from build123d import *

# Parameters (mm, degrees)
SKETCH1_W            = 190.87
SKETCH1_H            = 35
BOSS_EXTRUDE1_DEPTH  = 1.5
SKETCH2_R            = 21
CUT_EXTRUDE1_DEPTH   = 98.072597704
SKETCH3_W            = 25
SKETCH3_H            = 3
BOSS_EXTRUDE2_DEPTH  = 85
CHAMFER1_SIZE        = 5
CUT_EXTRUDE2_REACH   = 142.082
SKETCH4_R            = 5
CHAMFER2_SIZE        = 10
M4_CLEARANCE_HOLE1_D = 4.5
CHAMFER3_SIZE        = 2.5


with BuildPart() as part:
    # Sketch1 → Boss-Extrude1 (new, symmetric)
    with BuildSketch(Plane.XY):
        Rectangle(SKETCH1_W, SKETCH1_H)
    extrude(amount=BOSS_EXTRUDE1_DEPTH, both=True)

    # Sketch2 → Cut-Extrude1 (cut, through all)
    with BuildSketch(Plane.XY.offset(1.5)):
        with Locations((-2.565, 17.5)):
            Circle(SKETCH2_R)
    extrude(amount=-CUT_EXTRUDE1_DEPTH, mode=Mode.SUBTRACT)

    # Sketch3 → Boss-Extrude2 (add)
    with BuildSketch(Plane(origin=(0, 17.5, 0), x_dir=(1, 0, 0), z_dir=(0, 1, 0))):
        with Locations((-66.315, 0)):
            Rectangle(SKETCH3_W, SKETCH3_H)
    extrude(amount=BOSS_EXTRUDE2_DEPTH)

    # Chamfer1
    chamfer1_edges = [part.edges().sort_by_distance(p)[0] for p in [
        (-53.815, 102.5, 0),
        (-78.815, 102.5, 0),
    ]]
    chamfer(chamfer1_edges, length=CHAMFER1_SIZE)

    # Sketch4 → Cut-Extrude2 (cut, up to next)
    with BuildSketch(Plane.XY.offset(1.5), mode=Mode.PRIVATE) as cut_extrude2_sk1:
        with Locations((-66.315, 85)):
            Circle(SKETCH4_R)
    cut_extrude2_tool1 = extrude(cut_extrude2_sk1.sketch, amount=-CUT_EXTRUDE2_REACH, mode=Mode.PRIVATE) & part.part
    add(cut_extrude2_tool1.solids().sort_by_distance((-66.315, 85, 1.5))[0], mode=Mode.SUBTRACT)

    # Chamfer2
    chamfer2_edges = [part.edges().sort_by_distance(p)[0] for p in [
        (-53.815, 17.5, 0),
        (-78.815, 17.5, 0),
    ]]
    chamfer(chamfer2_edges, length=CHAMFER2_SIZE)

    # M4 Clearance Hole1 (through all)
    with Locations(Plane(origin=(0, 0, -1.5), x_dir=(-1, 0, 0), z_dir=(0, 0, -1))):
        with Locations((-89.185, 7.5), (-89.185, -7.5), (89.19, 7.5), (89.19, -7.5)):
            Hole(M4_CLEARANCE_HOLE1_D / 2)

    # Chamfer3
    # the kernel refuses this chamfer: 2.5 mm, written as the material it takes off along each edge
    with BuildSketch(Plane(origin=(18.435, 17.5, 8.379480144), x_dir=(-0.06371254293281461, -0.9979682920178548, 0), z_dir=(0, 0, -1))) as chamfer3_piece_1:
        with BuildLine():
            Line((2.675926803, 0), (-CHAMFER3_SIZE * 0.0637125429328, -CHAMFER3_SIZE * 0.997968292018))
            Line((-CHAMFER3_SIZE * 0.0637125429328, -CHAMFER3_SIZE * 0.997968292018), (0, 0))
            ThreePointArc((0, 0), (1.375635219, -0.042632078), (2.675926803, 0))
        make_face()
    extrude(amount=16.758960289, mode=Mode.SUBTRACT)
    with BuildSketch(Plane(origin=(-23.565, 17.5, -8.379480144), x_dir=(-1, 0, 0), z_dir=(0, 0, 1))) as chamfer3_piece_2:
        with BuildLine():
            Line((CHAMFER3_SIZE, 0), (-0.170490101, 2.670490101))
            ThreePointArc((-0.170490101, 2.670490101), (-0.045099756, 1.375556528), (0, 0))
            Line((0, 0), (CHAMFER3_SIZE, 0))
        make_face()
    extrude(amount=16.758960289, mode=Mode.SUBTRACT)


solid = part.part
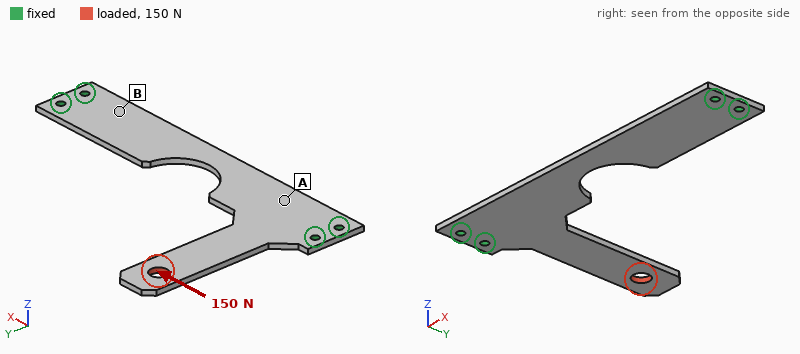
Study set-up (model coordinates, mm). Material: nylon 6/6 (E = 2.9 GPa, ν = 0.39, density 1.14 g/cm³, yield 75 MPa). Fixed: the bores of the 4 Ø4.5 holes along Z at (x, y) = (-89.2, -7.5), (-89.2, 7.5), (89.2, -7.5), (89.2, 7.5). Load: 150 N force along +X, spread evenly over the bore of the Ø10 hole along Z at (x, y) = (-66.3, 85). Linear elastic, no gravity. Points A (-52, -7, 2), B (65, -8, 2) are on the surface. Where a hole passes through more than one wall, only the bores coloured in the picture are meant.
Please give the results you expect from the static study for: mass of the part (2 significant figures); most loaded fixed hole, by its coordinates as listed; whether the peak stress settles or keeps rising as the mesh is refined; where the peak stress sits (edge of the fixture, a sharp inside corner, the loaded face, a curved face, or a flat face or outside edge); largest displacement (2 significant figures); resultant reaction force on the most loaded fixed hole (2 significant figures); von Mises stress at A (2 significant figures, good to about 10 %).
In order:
27 g
(-89.2, 7.5)
keeps rising
a sharp inside corner
2.7 mm
530 N
4.0 MPa
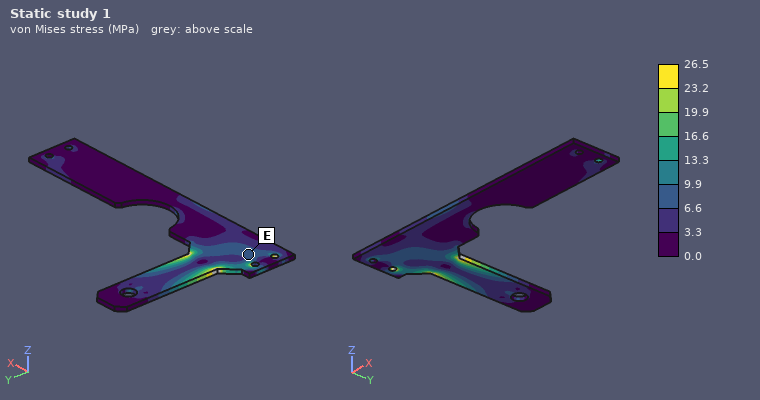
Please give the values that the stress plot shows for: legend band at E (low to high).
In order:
6.6 to 9.9 MPa
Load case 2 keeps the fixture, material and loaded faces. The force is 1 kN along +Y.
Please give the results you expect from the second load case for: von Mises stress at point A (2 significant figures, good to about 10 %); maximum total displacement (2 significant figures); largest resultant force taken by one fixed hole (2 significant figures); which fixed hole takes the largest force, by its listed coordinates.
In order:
5.1 MPa
1.5 mm
920 N
(-89.2, 7.5)
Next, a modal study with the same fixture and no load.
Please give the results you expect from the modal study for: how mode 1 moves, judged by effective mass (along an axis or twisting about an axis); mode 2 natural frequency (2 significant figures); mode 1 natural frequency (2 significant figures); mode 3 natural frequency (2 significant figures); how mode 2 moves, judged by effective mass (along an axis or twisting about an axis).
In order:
along Z
170 Hz
90 Hz
380 Hz
along Z
